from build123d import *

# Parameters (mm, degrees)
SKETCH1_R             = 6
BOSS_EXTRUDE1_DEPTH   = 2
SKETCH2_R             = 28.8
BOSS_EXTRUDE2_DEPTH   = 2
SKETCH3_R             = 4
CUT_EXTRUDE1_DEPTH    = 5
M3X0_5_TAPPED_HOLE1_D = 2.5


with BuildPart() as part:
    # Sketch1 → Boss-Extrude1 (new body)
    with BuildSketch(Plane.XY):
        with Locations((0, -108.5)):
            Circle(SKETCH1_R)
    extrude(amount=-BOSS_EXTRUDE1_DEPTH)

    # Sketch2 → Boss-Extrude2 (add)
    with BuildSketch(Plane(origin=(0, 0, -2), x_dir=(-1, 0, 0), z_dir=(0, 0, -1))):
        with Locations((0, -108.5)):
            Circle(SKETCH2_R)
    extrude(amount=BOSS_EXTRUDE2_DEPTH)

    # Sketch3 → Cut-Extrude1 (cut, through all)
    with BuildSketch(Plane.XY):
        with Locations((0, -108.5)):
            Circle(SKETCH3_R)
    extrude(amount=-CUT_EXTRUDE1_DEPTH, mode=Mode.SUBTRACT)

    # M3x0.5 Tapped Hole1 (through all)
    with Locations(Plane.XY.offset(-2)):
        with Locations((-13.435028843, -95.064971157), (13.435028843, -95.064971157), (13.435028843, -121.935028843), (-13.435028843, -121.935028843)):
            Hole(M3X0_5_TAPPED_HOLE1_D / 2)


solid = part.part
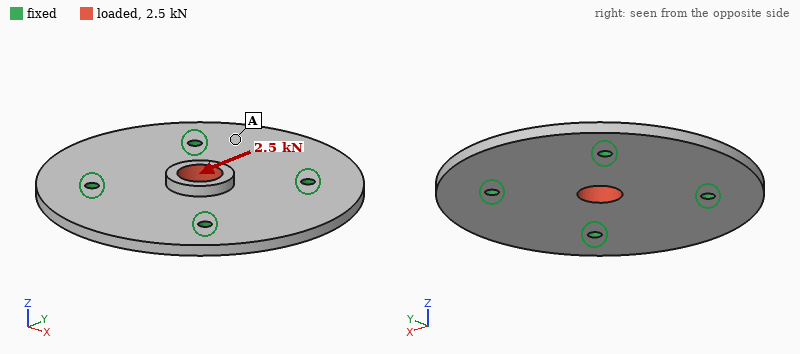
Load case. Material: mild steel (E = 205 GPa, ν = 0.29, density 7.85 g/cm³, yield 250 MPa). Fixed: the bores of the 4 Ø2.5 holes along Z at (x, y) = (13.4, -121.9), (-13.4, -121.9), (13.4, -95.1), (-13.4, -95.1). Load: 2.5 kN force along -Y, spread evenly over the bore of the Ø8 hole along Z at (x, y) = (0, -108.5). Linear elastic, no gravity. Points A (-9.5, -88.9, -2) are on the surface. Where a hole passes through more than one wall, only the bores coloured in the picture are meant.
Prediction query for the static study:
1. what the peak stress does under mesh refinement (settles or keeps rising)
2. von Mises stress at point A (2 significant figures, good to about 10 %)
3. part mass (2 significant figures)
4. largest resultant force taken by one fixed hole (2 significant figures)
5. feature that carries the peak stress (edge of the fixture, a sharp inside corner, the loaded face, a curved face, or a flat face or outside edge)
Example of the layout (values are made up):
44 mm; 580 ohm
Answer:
keeps rising; 11 MPa; 41 g; 650 N; edge of the fixture
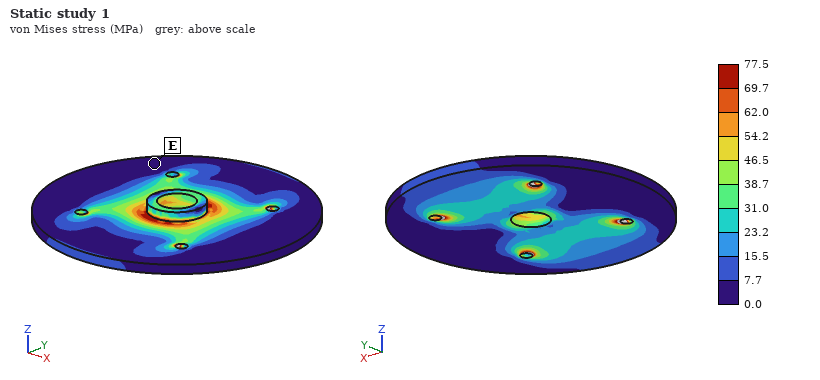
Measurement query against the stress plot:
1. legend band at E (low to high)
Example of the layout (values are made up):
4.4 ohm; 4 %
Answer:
0.0 to 7.7 MPa
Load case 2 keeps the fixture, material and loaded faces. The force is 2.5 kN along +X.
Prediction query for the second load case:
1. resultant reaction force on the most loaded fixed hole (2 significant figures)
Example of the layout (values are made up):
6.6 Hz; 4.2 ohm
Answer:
650 N
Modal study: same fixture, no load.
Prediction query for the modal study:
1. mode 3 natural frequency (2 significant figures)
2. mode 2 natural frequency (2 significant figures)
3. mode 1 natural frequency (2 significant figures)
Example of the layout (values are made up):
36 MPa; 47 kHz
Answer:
7200 Hz; 7200 Hz; 6500 Hz
